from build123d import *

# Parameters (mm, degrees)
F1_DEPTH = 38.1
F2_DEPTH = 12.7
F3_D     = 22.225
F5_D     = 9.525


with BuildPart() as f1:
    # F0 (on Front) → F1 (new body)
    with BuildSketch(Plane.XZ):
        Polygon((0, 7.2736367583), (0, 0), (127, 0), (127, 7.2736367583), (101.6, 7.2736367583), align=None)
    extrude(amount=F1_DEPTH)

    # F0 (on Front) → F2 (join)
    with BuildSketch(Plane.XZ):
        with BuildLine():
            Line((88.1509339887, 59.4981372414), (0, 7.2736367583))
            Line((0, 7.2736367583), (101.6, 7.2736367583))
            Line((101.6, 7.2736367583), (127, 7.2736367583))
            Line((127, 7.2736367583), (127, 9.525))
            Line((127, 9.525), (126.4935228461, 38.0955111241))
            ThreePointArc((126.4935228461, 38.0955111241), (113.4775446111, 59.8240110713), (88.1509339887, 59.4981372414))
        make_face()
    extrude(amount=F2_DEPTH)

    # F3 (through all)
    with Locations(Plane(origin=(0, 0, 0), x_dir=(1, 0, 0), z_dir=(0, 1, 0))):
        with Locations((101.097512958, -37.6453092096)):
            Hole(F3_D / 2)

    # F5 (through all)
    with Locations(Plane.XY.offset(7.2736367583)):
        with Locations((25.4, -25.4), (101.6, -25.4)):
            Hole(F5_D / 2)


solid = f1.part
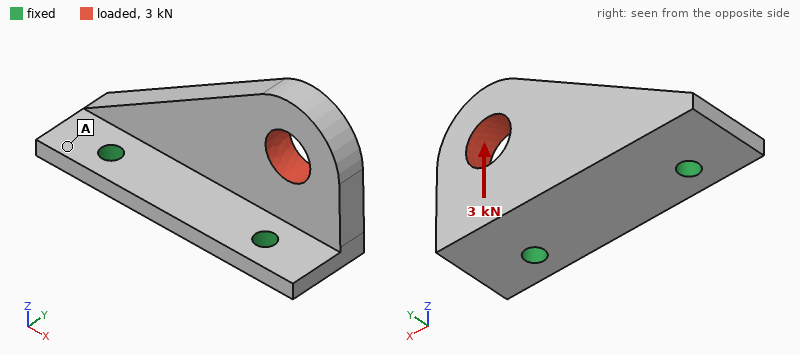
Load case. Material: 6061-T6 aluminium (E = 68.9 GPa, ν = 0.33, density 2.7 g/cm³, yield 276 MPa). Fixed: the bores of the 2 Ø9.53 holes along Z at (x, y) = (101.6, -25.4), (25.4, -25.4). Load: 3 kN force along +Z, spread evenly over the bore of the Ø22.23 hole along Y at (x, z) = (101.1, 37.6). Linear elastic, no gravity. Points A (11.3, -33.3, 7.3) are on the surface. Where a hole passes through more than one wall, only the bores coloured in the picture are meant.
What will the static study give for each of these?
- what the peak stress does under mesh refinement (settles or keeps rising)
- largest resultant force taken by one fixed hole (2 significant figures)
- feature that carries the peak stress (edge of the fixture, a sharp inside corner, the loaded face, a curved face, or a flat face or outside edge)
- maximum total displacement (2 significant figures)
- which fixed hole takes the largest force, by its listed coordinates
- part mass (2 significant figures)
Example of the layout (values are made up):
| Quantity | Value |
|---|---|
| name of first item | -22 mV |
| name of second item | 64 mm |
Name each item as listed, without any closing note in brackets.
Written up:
| Quantity | Value |
|---|---|
| what the peak stress does under mesh refinement | keeps rising |
| largest resultant force taken by one fixed hole | 2.9 kN |
| feature that carries the peak stress | edge of the fixture |
| maximum total displacement | 0.18 mm |
| which fixed hole takes the largest force, by its listed coordinates | (101.6, -25.4) |
| part mass | 230 g |
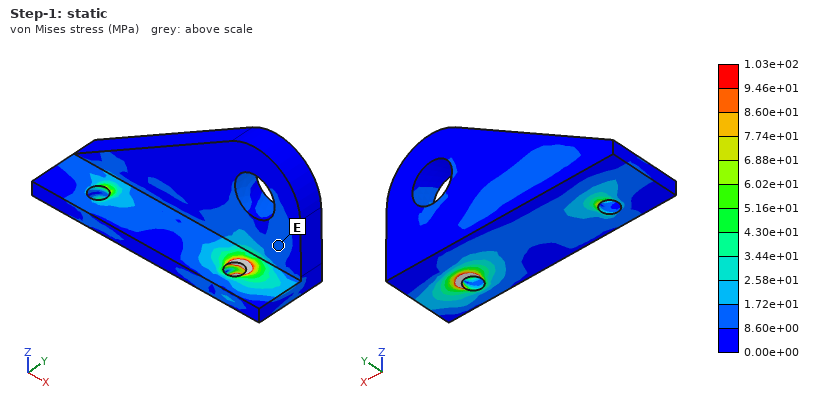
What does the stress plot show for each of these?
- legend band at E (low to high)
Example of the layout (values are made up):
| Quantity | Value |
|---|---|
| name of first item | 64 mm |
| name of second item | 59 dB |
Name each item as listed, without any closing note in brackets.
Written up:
| Quantity | Value |
|---|---|
| legend band at E | 8.60e+00 to 1.72e+01 MPa |
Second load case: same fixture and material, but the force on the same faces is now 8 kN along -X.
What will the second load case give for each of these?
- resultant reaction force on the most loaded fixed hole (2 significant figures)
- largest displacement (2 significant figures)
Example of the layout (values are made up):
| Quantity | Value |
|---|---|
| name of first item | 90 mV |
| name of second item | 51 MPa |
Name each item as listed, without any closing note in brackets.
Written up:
| Quantity | Value |
|---|---|
| resultant reaction force on the most loaded fixed hole | 5.6 kN |
| largest displacement | 0.13 mm |
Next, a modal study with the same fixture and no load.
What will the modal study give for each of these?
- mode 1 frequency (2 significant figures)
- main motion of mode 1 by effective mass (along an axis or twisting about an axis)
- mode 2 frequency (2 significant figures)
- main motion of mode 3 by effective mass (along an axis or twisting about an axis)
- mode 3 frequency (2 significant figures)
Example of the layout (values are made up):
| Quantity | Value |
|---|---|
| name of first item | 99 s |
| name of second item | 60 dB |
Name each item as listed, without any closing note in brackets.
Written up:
| Quantity | Value |
|---|---|
| mode 1 frequency | 1500 Hz |
| main motion of mode 1 by effective mass | along Y |
| mode 2 frequency | 4200 Hz |
| main motion of mode 3 by effective mass | along Z |
| mode 3 frequency | 5500 Hz |
